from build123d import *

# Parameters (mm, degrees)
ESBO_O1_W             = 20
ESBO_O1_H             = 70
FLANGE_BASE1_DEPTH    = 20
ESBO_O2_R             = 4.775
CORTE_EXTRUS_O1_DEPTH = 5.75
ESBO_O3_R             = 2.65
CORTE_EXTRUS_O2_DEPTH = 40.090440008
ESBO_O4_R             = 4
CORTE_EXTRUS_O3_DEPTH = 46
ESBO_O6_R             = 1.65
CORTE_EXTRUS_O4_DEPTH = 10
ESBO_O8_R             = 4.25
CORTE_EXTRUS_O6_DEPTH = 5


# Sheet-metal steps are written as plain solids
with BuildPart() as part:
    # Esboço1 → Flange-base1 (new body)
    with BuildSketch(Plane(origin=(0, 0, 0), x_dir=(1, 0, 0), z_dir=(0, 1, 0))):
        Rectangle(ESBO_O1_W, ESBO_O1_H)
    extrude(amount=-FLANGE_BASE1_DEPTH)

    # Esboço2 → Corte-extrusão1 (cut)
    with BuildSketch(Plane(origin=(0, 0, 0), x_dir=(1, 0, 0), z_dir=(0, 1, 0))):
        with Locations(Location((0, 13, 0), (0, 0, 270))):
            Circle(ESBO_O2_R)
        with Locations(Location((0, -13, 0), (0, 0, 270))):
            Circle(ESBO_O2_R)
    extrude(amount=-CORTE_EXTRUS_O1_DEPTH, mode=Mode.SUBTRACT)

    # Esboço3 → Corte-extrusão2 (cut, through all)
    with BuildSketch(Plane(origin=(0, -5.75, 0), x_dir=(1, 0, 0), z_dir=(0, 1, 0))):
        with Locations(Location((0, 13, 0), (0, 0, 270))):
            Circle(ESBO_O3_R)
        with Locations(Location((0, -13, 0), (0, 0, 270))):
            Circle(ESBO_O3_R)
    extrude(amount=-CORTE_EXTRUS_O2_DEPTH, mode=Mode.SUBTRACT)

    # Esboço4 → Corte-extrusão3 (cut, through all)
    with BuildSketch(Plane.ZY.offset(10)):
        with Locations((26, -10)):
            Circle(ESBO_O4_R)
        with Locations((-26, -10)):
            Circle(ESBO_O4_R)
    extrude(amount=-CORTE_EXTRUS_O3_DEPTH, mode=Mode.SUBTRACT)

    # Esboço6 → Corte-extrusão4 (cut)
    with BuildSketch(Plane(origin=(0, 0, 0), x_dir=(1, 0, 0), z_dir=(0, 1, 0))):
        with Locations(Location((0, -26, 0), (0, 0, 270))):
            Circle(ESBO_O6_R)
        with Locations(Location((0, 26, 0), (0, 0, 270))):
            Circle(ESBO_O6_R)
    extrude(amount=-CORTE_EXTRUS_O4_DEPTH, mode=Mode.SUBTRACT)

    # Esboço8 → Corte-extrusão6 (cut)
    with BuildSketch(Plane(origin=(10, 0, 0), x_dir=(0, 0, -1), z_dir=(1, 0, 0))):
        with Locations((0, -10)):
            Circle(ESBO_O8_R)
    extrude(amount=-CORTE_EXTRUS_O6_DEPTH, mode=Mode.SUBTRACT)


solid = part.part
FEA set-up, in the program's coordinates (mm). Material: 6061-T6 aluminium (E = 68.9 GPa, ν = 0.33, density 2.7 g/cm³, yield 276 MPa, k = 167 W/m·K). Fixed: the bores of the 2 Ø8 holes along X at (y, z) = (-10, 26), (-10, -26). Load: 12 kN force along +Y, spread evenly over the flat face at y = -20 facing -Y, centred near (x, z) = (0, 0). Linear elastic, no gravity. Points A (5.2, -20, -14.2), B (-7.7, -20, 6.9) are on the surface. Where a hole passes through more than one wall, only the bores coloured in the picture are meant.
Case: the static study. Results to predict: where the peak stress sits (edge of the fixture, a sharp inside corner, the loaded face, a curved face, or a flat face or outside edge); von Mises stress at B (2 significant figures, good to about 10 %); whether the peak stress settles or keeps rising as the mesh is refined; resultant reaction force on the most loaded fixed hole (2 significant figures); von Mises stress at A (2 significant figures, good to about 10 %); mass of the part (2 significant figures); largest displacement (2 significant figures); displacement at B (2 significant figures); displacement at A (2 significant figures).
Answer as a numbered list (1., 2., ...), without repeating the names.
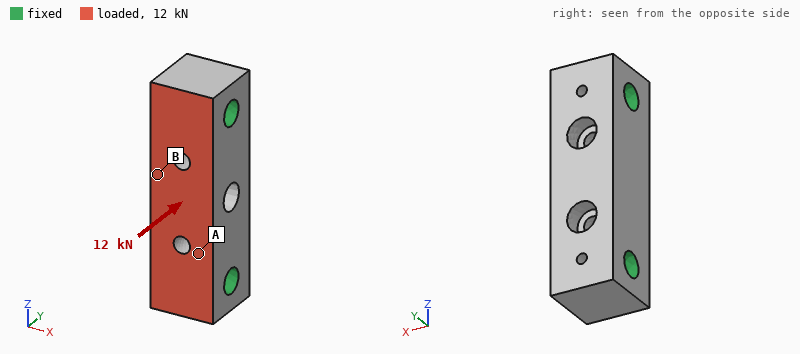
1. edge of the fixture
2. 19 MPa
3. keeps rising
4. 6.0 kN
5. 7.2 MPa
6. 65 g
7. 12 µm
8. 11 µm
9. 7.7 µm
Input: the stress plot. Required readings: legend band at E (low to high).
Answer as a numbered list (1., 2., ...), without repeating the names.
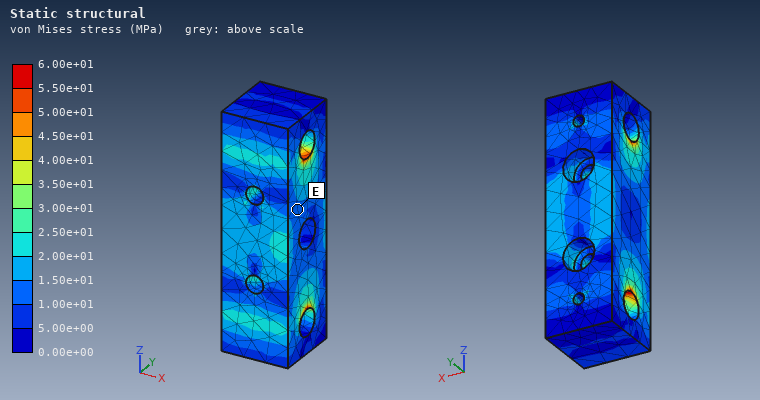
1. 1.00e+01 to 1.50e+01 MPa
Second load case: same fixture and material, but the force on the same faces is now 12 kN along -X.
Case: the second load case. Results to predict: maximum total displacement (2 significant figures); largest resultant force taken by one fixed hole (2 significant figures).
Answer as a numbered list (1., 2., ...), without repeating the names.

1. 27 µm
2. 6.0 kN
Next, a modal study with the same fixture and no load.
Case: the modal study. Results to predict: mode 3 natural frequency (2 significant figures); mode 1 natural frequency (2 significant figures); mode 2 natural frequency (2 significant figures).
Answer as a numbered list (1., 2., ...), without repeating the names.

1. 27 kHz
2. 22 kHz
3. 22 kHz
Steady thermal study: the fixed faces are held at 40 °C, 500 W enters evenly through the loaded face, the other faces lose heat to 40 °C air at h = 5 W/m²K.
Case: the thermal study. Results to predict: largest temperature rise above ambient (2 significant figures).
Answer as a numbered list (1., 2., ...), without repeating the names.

1. 54 K
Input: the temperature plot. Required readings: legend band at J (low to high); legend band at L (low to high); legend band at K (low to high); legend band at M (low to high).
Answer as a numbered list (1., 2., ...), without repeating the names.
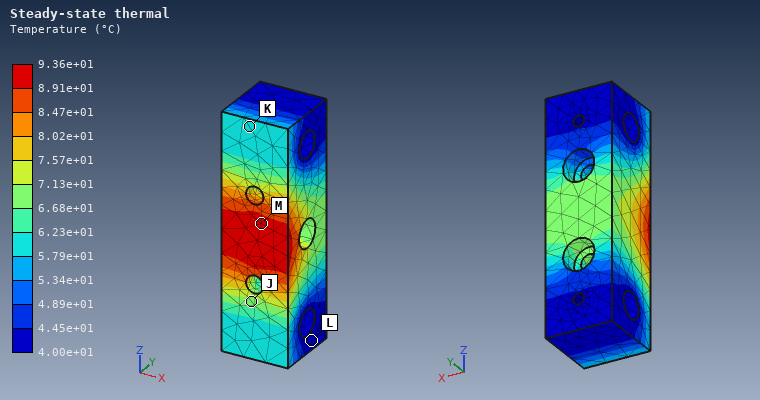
1. 6.68e+01 to 7.13e+01 °C
2. 4.00e+01 to 4.45e+01 °C
3. 5.79e+01 to 6.23e+01 °C
4. 8.91e+01 to 9.36e+01 °C
